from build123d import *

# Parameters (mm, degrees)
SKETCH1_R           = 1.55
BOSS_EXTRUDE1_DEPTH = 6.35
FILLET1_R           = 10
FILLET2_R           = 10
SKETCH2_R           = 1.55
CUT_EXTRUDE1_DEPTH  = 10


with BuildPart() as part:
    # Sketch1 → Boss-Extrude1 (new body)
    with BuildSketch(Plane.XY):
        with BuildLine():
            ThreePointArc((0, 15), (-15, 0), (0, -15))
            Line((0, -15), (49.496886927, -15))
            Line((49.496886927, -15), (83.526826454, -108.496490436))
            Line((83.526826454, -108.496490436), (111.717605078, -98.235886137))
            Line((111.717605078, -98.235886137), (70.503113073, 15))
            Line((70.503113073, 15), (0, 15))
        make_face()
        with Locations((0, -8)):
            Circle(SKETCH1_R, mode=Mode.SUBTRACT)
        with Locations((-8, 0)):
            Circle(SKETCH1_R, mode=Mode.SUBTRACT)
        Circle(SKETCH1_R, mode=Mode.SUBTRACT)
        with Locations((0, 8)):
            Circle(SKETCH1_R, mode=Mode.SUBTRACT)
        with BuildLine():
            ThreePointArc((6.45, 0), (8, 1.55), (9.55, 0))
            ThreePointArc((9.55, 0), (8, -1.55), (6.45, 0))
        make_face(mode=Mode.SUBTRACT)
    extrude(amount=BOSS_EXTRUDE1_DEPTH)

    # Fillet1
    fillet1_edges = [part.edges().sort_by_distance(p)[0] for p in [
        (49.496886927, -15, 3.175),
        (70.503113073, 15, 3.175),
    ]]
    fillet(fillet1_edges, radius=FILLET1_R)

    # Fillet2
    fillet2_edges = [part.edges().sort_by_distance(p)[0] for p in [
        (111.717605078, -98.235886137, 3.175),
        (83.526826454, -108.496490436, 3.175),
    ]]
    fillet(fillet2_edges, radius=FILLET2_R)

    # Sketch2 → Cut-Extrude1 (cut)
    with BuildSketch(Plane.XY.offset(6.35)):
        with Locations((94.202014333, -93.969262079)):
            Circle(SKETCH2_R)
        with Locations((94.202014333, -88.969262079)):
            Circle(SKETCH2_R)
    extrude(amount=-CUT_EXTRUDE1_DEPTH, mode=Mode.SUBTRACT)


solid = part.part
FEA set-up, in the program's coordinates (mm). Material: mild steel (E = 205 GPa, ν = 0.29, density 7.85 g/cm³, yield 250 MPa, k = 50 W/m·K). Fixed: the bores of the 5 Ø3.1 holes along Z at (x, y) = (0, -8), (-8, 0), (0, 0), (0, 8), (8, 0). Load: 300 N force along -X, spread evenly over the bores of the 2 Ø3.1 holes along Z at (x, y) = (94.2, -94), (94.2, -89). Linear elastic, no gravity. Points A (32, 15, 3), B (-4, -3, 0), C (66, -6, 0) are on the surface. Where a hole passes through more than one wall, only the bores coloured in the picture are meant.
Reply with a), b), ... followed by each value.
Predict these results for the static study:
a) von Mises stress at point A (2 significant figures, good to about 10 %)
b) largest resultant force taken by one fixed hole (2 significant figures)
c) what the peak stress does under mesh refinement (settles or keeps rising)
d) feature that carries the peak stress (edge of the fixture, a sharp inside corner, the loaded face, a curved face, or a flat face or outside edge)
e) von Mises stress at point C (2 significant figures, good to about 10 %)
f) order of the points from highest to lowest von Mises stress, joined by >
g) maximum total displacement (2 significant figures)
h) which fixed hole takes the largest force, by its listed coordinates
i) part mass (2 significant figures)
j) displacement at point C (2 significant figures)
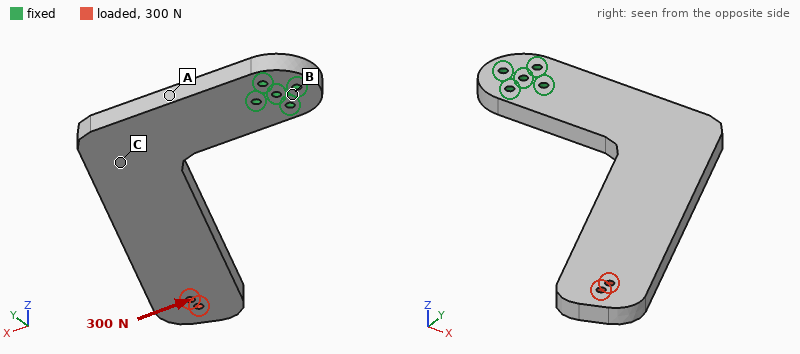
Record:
a) 28 MPa
b) 1.2 kN
c) keeps rising
d) edge of the fixture
e) 11 MPa
f) A > C > B
g) 0.10 mm
h) (0, -8)
i) 270 g
j) 0.022 mm
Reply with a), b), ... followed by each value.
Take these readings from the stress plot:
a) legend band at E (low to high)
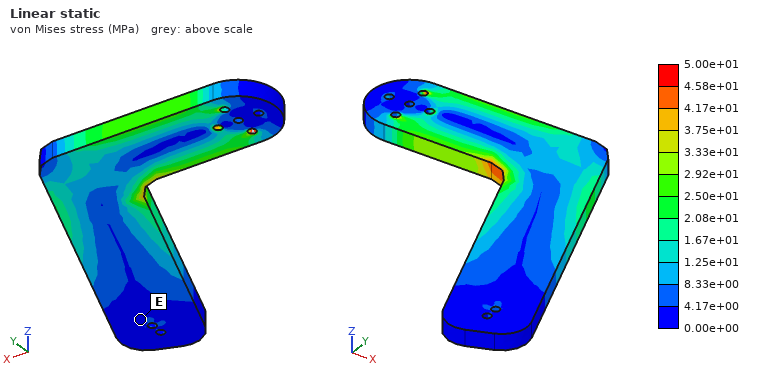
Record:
a) 0.00e+00 to 4.17e+00 MPa
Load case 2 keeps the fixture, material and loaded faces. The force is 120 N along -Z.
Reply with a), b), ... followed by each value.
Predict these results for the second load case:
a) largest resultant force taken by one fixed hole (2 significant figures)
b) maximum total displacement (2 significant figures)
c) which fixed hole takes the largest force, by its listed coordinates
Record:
a) 660 N
b) 0.82 mm
c) (8, 0)
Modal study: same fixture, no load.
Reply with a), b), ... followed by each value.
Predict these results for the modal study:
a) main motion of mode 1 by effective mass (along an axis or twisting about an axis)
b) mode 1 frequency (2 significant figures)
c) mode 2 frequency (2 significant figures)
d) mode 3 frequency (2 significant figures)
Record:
a) along Z
b) 250 Hz
c) 970 Hz
d) 1000 Hz
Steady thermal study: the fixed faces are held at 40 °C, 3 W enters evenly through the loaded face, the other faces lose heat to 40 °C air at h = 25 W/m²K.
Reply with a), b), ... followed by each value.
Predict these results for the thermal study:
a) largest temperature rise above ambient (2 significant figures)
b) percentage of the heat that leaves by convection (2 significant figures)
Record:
a) 20 K
b) 78 %
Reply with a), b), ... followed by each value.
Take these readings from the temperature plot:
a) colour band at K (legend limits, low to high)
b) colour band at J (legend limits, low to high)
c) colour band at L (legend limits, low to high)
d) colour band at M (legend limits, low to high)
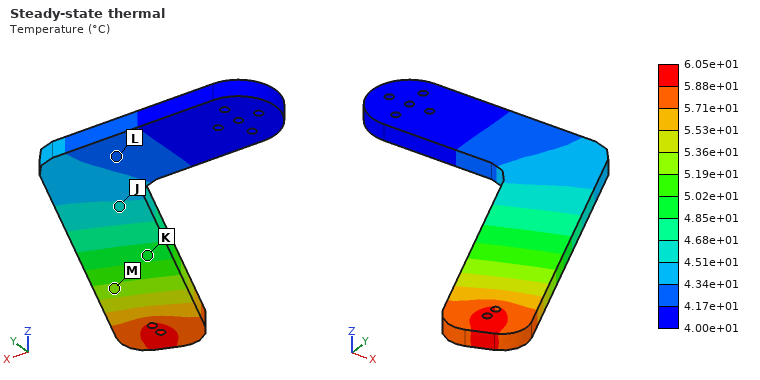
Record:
a) 4.85e+01 to 5.02e+01 °C
b) 4.51e+01 to 4.68e+01 °C
c) 4.17e+01 to 4.34e+01 °C
d) 5.19e+01 to 5.36e+01 °C
